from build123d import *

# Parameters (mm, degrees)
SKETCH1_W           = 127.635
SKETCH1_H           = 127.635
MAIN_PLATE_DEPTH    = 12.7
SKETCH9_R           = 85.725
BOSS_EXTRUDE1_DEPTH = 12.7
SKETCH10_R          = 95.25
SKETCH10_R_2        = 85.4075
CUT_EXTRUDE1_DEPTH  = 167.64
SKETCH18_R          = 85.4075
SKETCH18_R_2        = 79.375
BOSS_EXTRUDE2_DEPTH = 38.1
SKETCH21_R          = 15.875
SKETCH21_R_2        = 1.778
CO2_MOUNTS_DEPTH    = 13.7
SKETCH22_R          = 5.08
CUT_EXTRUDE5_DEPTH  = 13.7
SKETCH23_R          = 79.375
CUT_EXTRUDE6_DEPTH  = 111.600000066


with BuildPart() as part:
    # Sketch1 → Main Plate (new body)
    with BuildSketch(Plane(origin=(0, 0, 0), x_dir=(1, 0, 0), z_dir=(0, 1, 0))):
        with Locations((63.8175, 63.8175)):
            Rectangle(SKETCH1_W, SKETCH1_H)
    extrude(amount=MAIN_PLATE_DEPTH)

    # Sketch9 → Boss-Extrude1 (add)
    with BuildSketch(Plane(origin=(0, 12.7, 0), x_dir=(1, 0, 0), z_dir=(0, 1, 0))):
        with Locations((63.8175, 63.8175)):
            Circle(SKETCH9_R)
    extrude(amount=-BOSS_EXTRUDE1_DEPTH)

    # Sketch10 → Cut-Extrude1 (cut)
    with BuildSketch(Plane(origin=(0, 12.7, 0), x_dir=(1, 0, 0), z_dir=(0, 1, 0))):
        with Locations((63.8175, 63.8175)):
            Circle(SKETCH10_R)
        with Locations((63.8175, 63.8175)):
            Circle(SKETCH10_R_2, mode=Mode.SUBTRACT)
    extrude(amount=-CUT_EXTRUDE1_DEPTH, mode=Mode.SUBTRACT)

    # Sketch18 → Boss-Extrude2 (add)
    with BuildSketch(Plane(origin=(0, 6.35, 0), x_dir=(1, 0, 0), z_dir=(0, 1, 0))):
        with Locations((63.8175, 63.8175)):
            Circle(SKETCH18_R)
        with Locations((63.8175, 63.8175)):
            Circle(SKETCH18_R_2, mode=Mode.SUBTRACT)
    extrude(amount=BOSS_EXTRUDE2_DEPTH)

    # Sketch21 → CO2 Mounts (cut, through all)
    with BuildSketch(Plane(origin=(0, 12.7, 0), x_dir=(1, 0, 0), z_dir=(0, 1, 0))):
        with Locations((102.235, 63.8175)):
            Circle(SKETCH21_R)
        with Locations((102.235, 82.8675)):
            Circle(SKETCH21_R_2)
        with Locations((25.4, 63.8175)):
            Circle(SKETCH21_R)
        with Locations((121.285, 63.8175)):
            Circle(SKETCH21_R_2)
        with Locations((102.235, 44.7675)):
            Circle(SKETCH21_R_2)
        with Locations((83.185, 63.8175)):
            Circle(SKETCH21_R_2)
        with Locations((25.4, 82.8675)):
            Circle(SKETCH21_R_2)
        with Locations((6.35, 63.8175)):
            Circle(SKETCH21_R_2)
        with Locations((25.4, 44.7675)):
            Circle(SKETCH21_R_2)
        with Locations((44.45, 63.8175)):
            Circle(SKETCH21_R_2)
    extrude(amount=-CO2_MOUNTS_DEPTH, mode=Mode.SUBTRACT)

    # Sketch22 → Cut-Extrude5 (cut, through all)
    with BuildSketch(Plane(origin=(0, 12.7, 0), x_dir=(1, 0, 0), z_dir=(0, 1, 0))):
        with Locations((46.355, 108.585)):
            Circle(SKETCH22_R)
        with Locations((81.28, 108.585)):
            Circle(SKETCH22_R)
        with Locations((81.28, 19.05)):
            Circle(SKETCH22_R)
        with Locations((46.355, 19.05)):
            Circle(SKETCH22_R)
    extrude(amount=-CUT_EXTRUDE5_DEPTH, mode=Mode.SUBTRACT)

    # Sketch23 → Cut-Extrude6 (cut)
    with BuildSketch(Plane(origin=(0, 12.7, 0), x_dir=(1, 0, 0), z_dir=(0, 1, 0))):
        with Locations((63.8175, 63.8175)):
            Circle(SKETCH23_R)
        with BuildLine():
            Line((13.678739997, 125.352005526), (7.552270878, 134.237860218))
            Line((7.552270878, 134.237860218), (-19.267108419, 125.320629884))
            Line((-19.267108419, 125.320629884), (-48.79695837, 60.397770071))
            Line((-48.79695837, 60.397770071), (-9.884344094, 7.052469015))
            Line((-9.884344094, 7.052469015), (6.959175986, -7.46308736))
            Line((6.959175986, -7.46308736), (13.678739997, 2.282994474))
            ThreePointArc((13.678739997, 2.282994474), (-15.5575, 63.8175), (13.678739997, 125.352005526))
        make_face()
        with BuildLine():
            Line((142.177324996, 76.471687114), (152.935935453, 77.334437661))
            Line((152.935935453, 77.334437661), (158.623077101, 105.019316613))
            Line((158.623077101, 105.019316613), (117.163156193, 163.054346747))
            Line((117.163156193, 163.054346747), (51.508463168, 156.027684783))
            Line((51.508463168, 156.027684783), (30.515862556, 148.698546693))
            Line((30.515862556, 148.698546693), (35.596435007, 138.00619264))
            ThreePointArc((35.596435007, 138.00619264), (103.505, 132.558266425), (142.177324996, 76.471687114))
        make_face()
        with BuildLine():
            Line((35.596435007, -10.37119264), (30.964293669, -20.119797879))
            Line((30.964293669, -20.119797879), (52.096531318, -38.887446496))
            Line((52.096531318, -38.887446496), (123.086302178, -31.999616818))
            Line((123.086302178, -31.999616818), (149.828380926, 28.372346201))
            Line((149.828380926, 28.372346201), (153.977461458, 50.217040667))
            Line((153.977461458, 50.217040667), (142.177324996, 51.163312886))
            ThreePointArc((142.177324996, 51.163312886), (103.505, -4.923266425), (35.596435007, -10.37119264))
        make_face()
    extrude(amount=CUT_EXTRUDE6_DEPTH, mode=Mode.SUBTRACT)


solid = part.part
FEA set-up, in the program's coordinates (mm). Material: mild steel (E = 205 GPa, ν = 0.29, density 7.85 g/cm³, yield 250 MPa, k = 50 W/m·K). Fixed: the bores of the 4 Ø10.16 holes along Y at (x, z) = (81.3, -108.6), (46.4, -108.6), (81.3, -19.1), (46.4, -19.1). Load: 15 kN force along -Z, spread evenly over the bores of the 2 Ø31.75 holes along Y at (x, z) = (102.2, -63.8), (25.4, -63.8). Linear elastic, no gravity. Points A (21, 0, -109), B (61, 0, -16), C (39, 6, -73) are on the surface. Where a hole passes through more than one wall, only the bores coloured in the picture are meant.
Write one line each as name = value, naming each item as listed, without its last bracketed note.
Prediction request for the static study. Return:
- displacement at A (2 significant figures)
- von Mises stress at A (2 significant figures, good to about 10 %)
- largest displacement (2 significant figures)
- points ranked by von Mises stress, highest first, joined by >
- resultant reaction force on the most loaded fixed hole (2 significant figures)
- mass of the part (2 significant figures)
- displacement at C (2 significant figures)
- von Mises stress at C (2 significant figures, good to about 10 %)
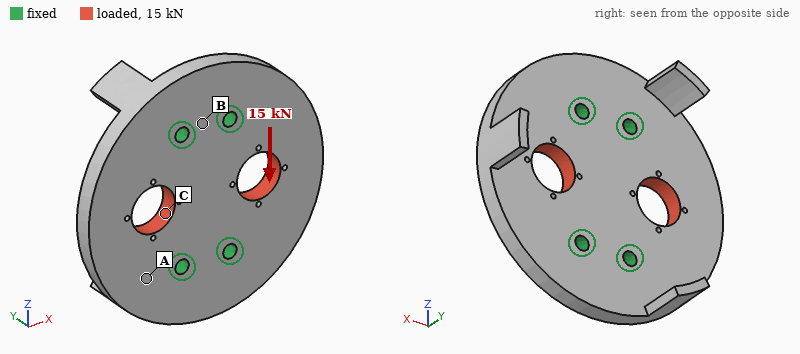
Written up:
displacement at A = 1.5 µm
von Mises stress at A = 4.7 MPa
largest displacement = 3.0 µm
points ranked by von Mises stress, highest first, joined by > = C > A > B
resultant reaction force on the most loaded fixed hole = 3.8 kN
mass of the part = 2.2 kg
displacement at C = 1.3 µm
von Mises stress at C = 10 MPa
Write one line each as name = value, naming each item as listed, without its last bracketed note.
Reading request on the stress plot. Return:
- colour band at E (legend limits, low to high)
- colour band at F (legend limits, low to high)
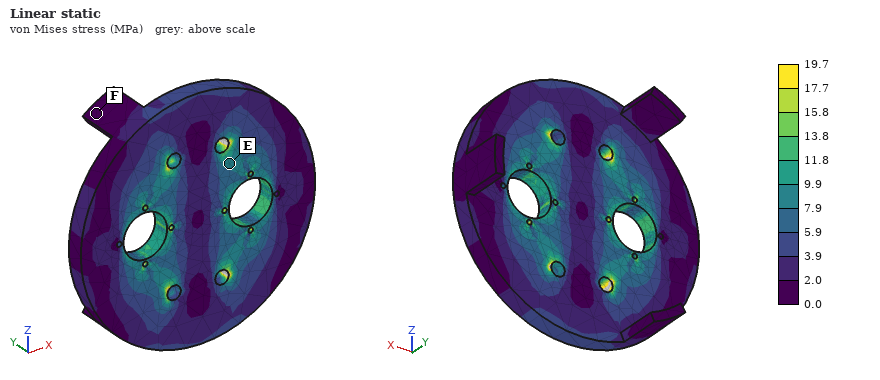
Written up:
colour band at E = 7.9 to 9.9 MPa
colour band at F = 0.0 to 2.0 MPa
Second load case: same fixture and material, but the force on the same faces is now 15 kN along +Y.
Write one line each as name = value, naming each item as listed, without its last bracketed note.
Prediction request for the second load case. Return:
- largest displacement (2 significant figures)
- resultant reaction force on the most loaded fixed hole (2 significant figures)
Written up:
largest displacement = 51 µm
resultant reaction force on the most loaded fixed hole = 3.8 kN
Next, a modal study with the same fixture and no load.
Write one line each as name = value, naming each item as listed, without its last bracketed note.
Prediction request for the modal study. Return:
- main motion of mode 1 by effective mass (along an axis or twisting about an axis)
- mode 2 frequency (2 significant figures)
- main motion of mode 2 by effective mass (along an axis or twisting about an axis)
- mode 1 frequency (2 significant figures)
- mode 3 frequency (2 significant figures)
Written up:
main motion of mode 1 by effective mass = along Y
mode 2 frequency = 2400 Hz
main motion of mode 2 by effective mass = along Y
mode 1 frequency = 2100 Hz
mode 3 frequency = 3600 Hz
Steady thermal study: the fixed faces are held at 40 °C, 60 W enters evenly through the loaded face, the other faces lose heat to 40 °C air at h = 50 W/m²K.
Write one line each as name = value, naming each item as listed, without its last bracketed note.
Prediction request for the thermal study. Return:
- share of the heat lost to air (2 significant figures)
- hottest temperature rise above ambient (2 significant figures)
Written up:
share of the heat lost to air = 29 %
hottest temperature rise above ambient = 17 K
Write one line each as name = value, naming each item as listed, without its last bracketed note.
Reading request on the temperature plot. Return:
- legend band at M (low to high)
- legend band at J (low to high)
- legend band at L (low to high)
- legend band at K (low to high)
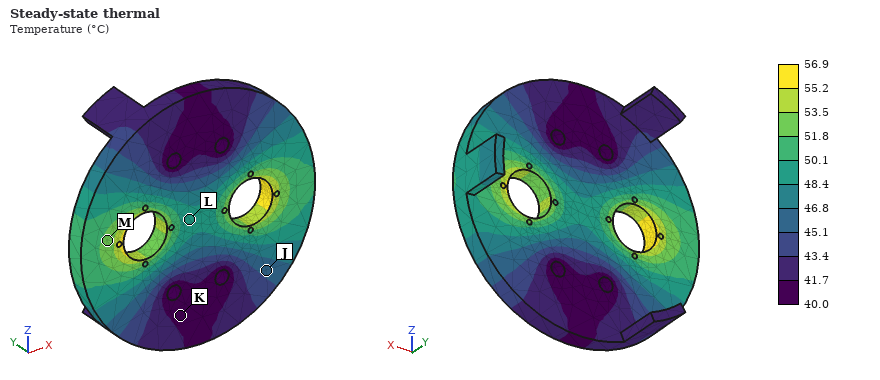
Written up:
legend band at M = 51.8 to 53.5 °C
legend band at J = 45.1 to 46.8 °C
legend band at L = 48.4 to 50.1 °C
legend band at K = 40.0 to 41.7 °C
